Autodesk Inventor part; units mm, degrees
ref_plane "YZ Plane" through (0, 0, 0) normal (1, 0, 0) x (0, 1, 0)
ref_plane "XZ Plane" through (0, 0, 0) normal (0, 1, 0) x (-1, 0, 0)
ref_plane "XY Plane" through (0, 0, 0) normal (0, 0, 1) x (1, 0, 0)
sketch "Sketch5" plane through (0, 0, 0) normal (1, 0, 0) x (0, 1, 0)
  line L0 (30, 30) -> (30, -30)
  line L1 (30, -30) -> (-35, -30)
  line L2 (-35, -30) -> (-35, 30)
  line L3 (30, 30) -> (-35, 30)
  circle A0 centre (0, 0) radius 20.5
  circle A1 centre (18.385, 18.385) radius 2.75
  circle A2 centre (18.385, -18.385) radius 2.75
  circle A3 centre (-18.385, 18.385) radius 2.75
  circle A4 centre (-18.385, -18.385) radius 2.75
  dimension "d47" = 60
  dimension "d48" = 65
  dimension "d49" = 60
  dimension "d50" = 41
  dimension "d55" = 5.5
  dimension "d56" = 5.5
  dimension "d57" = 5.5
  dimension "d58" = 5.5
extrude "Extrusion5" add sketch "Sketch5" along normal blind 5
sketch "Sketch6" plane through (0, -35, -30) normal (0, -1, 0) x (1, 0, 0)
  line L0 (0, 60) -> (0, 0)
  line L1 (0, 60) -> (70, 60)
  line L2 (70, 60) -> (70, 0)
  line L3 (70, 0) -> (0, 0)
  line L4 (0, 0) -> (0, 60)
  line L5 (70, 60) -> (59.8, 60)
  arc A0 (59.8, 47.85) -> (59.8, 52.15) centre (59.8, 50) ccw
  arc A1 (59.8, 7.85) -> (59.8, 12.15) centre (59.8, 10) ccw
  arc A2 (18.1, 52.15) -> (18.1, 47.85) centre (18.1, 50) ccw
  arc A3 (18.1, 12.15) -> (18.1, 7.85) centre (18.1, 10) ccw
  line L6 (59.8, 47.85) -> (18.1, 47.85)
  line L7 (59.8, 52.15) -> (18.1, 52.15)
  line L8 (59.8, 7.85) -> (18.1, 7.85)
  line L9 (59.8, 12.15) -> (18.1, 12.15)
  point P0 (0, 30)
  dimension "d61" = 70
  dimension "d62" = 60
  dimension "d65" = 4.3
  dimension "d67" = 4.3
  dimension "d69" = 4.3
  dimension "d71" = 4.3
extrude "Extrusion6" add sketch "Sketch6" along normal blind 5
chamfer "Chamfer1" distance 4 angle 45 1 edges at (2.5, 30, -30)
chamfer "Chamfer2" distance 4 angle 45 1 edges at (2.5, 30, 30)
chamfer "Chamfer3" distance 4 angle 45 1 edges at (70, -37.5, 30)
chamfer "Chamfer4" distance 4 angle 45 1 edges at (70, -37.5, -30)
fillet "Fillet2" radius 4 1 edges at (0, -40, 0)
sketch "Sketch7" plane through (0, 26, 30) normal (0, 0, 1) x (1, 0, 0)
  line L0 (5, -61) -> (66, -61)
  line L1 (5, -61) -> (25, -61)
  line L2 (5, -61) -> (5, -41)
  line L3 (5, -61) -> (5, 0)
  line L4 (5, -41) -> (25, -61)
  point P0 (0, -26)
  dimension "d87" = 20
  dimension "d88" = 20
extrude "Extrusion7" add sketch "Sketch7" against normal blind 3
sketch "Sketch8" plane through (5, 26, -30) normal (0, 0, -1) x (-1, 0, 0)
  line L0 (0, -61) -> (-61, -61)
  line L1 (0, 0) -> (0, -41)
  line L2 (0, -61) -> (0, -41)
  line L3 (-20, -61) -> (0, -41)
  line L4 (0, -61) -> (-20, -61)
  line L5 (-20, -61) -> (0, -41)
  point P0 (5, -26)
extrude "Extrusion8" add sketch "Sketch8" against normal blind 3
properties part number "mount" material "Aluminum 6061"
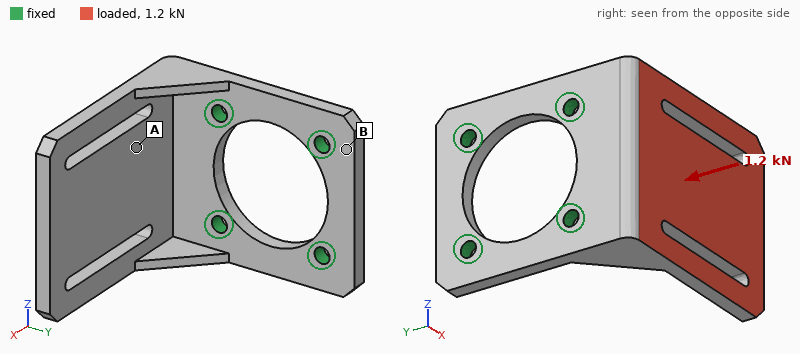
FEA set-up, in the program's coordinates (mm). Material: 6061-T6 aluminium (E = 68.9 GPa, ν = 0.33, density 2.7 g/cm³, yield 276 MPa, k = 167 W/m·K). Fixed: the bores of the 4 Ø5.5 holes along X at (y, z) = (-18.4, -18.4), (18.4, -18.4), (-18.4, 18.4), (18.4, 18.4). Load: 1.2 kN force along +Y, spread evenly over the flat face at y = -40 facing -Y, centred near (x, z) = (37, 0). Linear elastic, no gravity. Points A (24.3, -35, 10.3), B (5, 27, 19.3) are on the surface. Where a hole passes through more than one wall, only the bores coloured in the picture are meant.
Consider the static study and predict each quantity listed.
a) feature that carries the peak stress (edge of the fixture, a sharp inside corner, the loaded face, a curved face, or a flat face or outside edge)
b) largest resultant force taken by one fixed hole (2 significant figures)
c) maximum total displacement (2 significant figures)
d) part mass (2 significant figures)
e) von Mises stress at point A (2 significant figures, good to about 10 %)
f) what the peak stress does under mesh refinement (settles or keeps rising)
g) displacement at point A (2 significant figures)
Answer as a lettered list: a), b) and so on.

a) edge of the fixture
b) 520 N
c) 1.4 mm
d) 87 g
e) 58 MPa
f) keeps rising
g) 0.32 mm
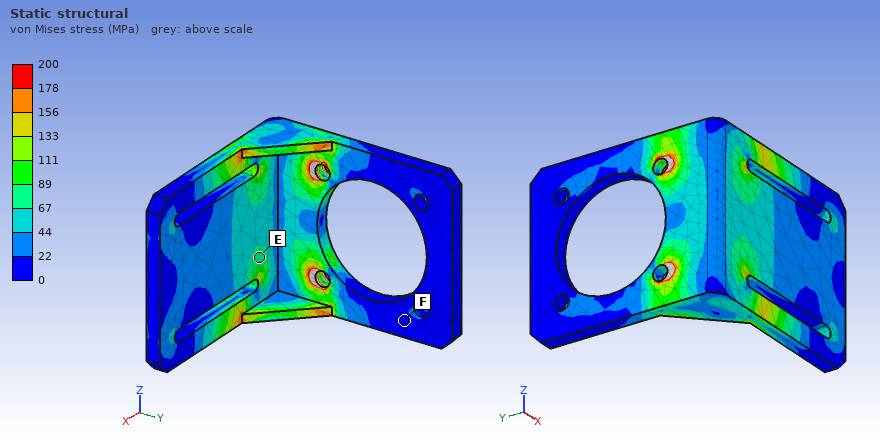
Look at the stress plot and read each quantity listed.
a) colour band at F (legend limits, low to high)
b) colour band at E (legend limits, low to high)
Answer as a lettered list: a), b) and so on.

a) 0 to 22 MPa
b) 67 to 89 MPa
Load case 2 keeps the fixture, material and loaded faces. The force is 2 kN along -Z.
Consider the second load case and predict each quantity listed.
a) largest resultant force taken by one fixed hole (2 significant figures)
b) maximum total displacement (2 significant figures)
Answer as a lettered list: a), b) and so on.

a) 2.1 kN
b) 0.34 mm
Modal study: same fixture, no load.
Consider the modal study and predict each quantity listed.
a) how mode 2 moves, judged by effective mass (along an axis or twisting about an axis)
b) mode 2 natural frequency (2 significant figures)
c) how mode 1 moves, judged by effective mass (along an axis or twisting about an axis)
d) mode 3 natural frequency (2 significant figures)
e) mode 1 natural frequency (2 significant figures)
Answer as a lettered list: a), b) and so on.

a) along Z
b) 1800 Hz
c) along Y
d) 3100 Hz
e) 840 Hz
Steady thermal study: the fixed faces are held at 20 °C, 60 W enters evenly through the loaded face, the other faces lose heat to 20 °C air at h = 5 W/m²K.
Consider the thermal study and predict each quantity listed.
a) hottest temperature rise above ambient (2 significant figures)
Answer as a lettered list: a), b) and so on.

a) 63 K
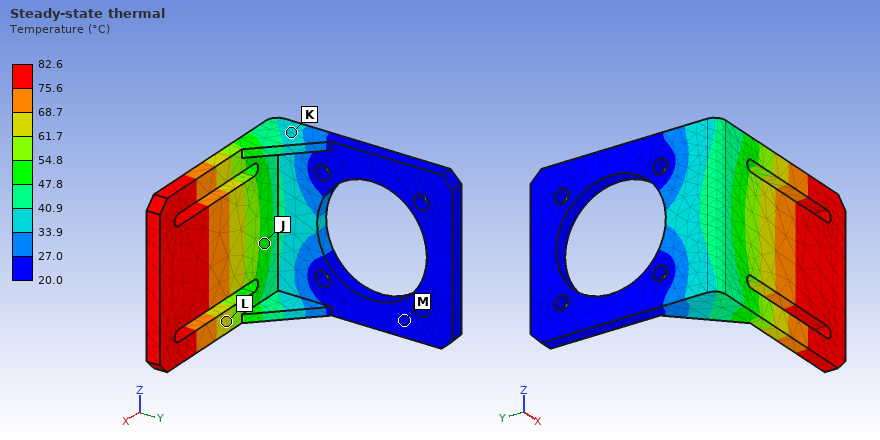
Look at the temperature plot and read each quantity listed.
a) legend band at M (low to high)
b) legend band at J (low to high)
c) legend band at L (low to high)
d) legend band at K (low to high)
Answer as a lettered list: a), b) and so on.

a) 20.0 to 27.0 °C
b) 47.8 to 54.8 °C
c) 61.7 to 68.7 °C
d) 33.9 to 40.9 °C
